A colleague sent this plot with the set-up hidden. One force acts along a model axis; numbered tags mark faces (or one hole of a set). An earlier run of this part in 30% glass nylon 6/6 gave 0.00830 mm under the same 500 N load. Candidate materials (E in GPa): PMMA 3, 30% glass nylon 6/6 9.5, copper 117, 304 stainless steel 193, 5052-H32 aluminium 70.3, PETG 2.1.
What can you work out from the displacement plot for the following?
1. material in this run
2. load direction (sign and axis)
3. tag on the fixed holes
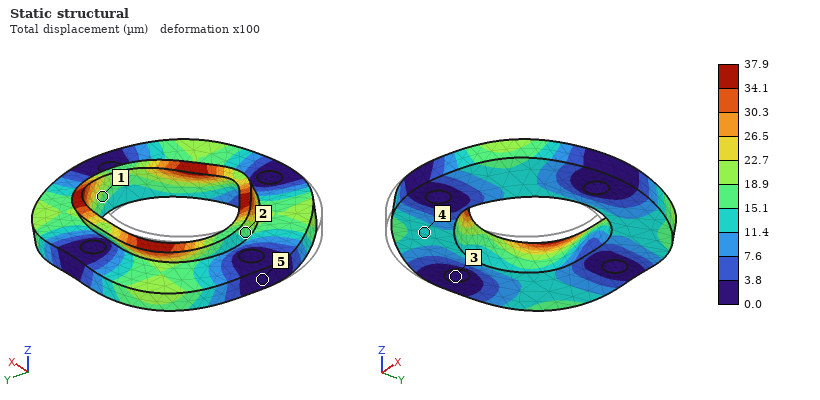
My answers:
PETG
+Y
3
